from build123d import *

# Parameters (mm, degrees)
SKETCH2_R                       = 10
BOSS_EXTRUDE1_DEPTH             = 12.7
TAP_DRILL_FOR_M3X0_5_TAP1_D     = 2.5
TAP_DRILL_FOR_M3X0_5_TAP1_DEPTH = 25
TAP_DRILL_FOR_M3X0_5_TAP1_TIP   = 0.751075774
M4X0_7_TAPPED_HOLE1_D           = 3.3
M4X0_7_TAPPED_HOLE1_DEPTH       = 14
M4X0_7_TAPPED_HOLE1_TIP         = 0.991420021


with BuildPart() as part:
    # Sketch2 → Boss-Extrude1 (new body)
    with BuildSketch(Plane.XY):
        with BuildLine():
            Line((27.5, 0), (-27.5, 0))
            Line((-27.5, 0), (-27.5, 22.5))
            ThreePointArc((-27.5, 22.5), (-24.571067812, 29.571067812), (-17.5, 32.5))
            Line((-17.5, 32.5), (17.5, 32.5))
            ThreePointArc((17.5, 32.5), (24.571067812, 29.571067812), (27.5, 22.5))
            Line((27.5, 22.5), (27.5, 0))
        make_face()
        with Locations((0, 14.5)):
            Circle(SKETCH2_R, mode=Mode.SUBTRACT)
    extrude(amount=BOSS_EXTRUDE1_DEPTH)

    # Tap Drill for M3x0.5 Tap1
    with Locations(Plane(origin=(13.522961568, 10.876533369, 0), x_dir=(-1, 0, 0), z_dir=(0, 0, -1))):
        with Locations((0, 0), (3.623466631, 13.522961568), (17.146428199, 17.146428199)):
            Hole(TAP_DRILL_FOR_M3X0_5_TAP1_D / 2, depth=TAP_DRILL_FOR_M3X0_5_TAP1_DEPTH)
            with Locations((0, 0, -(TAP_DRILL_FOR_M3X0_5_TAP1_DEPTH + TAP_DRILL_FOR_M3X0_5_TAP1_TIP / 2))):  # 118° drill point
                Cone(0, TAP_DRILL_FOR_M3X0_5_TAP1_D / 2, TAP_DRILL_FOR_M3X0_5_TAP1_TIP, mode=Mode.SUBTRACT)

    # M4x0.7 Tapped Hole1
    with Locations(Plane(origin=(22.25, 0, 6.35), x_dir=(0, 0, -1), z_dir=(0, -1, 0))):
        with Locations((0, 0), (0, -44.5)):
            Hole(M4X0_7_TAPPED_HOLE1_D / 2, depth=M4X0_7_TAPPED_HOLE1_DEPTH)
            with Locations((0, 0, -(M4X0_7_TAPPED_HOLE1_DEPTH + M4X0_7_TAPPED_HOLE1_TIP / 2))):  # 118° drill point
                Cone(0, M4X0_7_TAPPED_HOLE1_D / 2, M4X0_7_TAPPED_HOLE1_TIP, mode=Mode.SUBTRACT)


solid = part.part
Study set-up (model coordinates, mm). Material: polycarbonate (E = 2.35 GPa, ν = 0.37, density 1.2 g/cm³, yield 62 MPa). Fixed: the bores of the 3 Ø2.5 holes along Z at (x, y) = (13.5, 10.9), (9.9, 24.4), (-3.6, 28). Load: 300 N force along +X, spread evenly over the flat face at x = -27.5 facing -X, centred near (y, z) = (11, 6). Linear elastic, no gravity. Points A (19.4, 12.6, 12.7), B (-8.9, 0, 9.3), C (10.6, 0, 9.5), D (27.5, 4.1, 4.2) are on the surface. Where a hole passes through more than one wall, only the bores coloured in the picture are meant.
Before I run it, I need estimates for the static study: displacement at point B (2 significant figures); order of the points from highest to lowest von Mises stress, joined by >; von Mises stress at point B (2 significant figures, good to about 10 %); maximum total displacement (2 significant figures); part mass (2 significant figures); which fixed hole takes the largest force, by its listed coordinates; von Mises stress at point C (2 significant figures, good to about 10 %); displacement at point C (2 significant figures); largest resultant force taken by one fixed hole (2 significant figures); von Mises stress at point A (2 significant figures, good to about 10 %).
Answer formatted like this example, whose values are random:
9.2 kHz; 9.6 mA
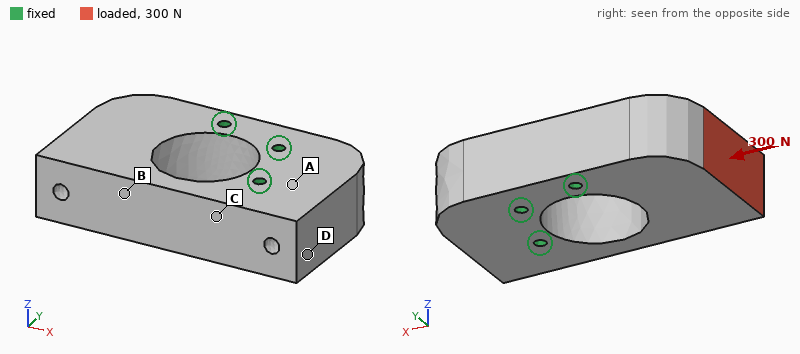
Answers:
52 µm; B > C > A > D; 3.6 MPa; 82 µm; 21 g; (13.5, 10.9); 2.4 MPa; 30 µm; 240 N; 1.0 MPa
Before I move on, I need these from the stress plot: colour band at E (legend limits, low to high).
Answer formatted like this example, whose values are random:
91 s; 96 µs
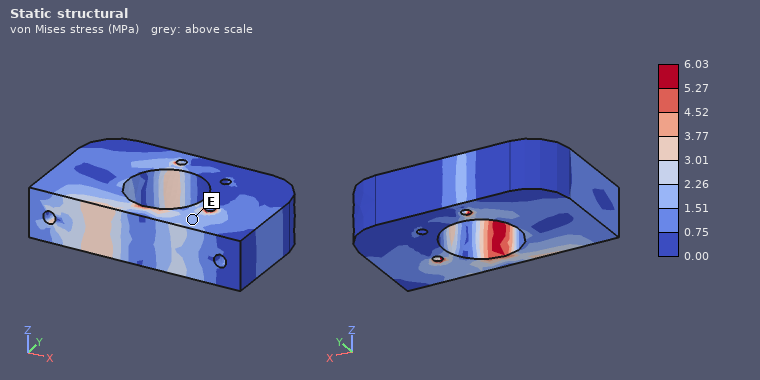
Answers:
1.51 to 2.26 MPa
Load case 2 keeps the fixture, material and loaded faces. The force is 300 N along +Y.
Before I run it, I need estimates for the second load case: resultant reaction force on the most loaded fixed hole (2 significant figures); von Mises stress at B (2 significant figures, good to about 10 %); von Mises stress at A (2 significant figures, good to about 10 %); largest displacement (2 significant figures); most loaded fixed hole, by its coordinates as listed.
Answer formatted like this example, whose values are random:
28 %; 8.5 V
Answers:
430 N; 4.2 MPa; 1.5 MPa; 0.16 mm; (-3.6, 28)
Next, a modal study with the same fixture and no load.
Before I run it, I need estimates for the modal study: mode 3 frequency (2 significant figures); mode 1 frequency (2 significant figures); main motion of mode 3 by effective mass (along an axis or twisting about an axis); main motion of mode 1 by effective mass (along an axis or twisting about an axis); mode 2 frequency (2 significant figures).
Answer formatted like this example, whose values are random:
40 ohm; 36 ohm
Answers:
4500 Hz; 2000 Hz; twisting about X; along Z; 3000 Hz
